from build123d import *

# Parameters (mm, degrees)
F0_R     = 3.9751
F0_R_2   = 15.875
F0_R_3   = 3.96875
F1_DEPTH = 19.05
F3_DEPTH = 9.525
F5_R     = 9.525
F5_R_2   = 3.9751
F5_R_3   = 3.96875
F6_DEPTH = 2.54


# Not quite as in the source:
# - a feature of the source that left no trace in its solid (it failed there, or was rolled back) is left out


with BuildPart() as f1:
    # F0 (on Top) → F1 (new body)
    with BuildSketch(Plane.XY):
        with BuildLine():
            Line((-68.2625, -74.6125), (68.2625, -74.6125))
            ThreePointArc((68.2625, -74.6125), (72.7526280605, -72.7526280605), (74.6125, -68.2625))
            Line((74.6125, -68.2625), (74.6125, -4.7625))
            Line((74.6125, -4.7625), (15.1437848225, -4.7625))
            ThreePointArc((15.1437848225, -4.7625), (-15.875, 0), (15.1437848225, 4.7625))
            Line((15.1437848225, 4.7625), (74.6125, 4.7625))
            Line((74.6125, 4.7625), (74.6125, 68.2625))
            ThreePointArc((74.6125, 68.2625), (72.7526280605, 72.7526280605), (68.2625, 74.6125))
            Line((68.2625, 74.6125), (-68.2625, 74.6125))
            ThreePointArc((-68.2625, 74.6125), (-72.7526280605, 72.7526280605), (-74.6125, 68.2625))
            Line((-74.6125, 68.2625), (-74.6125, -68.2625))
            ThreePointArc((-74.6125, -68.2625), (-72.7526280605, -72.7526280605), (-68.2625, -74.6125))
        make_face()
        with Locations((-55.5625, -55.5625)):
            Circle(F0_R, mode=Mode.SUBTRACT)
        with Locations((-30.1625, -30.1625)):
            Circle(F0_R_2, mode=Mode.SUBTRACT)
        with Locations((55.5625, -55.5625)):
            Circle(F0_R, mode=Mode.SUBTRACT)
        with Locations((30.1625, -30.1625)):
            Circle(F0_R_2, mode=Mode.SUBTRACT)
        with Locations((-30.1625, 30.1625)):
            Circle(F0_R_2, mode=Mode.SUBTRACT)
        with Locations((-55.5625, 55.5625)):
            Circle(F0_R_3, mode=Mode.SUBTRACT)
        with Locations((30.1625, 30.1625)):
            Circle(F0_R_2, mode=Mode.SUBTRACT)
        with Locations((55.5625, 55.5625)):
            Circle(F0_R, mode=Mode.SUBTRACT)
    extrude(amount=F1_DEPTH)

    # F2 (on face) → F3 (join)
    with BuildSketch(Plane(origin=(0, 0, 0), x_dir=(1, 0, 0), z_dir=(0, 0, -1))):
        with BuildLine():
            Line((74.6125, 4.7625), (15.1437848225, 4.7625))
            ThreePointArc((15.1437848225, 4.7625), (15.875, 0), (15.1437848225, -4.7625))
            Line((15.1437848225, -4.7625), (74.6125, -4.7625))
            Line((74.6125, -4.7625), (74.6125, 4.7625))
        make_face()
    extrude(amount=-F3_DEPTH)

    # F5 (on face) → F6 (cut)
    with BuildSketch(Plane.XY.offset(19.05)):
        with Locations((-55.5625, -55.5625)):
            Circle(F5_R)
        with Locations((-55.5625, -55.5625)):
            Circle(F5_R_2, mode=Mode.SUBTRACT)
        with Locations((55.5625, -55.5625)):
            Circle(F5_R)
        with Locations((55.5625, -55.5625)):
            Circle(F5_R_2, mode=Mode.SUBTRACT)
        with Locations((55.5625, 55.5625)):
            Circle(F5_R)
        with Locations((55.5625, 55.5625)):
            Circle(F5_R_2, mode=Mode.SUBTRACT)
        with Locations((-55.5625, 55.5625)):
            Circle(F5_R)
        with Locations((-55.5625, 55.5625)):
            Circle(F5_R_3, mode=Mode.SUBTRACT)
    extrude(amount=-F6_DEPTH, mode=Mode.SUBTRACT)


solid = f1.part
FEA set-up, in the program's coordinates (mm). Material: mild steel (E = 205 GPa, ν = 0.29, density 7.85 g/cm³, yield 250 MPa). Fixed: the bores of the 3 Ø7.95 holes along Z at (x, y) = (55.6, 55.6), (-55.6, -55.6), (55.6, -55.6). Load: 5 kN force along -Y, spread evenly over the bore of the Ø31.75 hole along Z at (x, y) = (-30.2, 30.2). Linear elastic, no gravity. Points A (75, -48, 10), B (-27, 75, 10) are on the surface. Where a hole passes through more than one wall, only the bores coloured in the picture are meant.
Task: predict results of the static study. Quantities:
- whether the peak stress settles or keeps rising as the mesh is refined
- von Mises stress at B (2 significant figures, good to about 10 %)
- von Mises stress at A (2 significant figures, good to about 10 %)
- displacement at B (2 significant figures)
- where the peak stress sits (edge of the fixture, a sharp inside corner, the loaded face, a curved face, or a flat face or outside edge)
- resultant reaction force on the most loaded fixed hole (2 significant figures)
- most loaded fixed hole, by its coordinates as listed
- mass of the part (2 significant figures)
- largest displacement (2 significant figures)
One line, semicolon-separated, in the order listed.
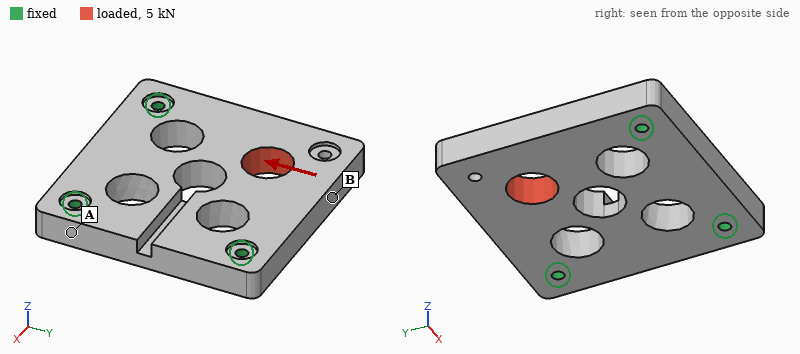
keeps rising; 4.6 MPa; 1.7 MPa; 3.0 µm; edge of the fixture; 3.2 kN; (-55.6, -55.6); 2.6 kg; 3.2 µm
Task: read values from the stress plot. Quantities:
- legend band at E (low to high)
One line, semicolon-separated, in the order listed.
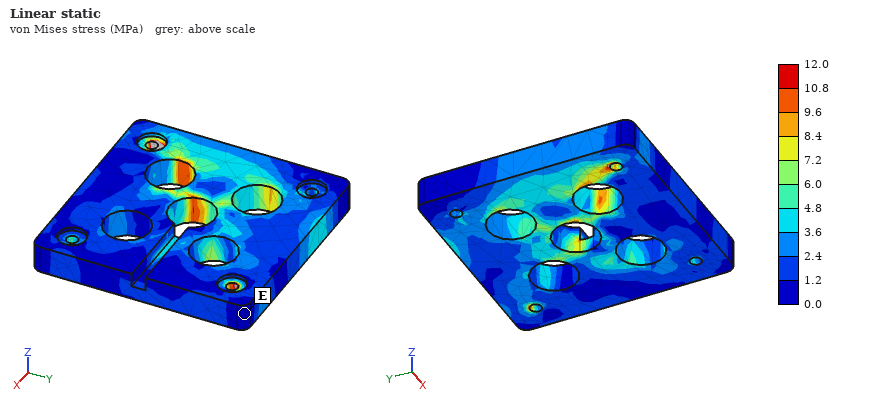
0.0 to 1.2 MPa
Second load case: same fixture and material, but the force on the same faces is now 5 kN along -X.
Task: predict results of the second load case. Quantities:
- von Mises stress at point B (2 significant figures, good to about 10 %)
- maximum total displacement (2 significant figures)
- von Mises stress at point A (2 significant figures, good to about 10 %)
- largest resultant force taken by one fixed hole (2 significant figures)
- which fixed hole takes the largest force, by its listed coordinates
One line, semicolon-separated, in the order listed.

1.5 MPa; 3.0 µm; 1.9 MPa; 3.2 kN; (55.6, 55.6)
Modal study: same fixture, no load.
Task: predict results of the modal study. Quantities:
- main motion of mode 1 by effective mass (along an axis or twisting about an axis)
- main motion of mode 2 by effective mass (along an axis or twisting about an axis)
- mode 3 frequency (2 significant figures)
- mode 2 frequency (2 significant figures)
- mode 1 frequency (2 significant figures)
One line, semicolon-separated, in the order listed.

along Z; along Z; 4700 Hz; 4000 Hz; 1400 Hz
